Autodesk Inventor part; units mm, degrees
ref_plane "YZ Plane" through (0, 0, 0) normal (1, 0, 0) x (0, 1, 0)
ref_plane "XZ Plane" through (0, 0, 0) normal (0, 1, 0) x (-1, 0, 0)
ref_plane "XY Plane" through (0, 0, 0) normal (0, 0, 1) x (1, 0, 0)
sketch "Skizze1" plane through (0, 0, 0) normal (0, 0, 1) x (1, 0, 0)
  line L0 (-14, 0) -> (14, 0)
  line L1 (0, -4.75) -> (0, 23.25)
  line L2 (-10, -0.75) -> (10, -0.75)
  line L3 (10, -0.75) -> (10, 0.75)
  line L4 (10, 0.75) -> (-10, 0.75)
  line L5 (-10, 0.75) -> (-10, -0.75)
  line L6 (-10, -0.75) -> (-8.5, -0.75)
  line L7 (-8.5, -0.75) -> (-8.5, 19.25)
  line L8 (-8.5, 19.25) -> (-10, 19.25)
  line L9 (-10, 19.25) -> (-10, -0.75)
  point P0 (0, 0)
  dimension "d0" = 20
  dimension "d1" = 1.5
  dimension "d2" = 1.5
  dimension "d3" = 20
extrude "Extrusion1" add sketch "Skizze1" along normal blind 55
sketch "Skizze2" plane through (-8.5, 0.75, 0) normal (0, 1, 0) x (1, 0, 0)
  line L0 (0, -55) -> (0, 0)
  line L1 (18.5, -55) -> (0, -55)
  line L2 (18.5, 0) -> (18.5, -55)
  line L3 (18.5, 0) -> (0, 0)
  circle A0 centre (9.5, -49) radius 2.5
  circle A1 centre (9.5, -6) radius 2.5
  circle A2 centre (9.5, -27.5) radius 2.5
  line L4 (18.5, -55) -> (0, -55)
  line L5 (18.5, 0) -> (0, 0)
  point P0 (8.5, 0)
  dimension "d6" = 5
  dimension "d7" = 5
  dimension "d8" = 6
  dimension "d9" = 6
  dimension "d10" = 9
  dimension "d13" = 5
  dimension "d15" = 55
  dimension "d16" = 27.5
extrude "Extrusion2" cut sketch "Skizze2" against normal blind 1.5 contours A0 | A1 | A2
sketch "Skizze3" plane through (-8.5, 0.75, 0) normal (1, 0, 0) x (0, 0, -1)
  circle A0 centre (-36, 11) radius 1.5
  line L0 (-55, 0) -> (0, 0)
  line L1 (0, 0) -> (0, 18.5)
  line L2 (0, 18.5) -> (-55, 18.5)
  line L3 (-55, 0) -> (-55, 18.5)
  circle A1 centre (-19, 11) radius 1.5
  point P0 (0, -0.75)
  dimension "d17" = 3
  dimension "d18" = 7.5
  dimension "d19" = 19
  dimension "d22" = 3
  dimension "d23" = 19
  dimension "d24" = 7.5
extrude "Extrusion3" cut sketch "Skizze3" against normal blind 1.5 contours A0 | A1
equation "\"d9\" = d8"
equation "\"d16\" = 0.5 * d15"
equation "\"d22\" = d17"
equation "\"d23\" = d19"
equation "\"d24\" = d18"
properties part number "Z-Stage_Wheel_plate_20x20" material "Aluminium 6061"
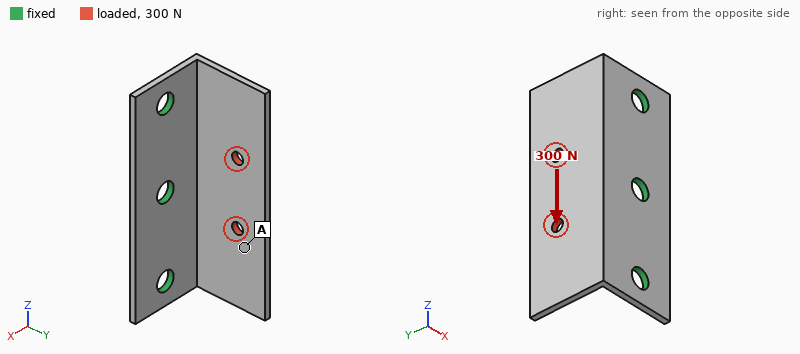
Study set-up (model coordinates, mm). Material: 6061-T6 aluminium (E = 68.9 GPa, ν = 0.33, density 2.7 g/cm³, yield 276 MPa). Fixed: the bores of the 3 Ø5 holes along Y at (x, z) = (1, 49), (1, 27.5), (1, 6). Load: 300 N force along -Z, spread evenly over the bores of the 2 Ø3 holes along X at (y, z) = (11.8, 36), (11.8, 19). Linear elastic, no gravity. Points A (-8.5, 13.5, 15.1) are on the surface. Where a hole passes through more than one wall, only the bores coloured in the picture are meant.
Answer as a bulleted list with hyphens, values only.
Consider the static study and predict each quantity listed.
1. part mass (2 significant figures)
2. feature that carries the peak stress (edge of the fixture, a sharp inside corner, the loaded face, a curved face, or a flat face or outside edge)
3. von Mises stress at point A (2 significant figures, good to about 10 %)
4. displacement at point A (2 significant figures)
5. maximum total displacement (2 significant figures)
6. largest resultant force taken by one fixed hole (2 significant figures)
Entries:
- 8.3 g
- a flat face or outside edge
- 13 MPa
- 0.050 mm
- 0.11 mm
- 130 N
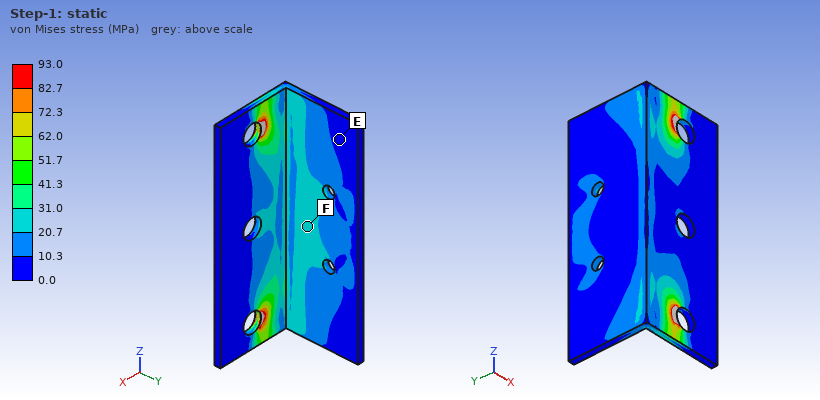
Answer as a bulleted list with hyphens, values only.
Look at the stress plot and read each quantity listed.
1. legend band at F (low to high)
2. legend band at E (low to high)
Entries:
- 20.7 to 31.0 MPa
- 0.0 to 10.3 MPa
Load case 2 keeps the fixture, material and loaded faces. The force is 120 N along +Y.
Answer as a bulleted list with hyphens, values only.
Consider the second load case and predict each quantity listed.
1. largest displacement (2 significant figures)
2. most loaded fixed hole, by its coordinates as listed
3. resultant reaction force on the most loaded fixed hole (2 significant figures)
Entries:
- 89 µm
- (1, 27.5)
- 48 N
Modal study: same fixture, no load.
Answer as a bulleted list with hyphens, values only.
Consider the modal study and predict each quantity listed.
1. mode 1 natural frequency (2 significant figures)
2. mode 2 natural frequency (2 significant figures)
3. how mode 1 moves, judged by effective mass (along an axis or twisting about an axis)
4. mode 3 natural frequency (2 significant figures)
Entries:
- 2000 Hz
- 3000 Hz
- along X
- 6300 Hz
